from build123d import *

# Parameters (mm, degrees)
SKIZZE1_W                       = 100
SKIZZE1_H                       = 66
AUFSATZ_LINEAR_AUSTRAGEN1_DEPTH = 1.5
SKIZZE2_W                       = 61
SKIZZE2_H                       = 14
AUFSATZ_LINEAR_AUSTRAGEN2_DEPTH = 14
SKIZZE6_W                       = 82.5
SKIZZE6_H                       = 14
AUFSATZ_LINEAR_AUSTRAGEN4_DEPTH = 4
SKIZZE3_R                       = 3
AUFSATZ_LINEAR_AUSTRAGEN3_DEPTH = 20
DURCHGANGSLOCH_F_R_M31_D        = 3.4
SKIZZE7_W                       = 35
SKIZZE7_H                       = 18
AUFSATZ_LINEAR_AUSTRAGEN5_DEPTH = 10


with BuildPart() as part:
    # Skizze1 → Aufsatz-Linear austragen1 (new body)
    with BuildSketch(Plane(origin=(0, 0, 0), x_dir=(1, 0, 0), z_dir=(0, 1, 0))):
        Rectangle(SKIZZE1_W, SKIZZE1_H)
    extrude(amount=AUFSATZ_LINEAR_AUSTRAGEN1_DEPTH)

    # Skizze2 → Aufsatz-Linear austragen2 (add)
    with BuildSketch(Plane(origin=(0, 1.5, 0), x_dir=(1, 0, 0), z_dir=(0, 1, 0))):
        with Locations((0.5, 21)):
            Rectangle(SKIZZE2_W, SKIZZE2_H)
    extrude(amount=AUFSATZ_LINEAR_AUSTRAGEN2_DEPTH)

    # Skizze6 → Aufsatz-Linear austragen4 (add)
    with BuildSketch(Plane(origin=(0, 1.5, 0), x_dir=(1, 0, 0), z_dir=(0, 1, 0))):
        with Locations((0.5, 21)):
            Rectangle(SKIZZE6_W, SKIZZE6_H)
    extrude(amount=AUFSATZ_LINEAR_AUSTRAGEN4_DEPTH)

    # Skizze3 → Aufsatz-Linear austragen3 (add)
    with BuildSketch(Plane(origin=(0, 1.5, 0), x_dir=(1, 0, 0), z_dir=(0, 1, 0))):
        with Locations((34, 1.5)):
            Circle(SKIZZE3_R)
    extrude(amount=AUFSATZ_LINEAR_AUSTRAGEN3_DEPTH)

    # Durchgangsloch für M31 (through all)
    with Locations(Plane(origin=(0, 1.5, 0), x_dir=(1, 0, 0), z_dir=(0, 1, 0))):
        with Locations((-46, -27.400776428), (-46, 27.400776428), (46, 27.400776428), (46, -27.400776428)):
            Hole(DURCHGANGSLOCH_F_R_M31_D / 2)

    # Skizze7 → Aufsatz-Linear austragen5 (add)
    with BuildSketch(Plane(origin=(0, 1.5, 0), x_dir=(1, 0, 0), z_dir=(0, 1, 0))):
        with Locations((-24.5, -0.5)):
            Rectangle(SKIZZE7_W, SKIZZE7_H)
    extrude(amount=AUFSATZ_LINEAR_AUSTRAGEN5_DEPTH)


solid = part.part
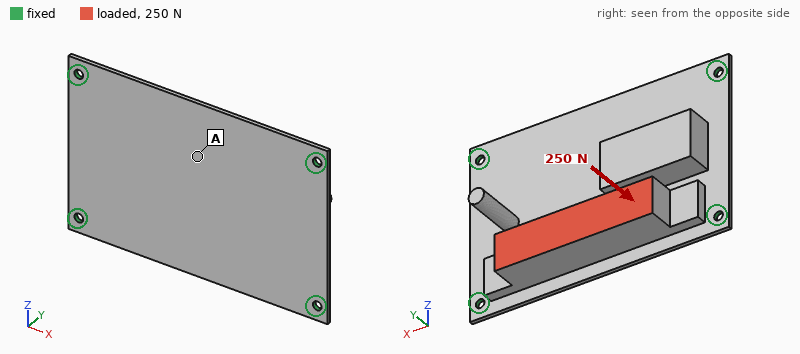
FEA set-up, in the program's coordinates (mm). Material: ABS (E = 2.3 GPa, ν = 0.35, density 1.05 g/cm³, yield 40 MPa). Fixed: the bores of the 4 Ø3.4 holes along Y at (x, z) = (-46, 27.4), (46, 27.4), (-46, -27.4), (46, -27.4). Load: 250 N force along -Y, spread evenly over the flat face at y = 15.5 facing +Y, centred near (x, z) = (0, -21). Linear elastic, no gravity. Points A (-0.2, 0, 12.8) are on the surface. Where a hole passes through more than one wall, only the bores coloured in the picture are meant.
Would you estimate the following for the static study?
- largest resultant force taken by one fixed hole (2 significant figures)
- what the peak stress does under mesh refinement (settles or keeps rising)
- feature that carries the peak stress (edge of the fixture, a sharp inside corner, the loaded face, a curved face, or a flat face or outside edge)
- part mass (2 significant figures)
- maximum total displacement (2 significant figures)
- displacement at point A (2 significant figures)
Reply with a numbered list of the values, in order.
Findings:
1. 210 N
2. keeps rising
3. edge of the fixture
4. 31 g
5. 1.3 mm
6. 1.1 mm
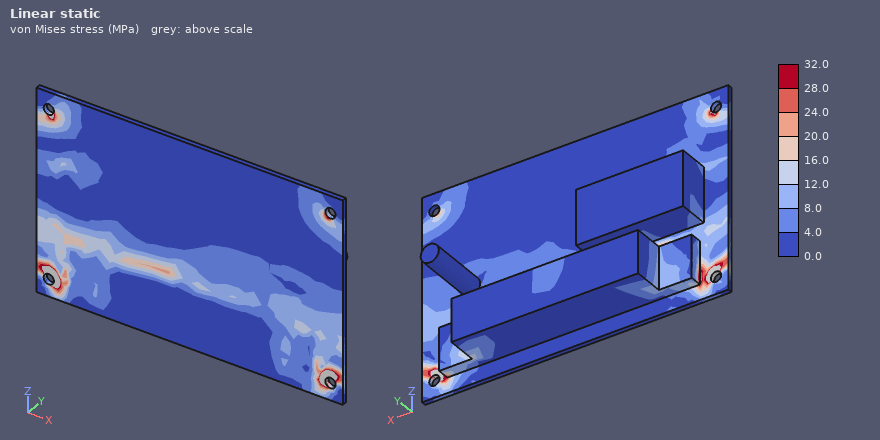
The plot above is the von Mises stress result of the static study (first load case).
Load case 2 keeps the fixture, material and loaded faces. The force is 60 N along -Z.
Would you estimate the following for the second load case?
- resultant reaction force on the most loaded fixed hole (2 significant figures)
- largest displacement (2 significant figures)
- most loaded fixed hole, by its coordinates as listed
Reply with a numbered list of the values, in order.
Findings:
1. 28 N
2. 0.75 mm
3. (-46, -27.4)
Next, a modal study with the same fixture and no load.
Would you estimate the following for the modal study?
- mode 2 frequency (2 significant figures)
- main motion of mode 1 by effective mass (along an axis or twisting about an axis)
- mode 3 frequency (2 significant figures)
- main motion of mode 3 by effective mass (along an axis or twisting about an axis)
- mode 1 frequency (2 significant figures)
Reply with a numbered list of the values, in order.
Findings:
1. 570 Hz
2. along Y
3. 760 Hz
4. twisting about Z
5. 320 Hz
